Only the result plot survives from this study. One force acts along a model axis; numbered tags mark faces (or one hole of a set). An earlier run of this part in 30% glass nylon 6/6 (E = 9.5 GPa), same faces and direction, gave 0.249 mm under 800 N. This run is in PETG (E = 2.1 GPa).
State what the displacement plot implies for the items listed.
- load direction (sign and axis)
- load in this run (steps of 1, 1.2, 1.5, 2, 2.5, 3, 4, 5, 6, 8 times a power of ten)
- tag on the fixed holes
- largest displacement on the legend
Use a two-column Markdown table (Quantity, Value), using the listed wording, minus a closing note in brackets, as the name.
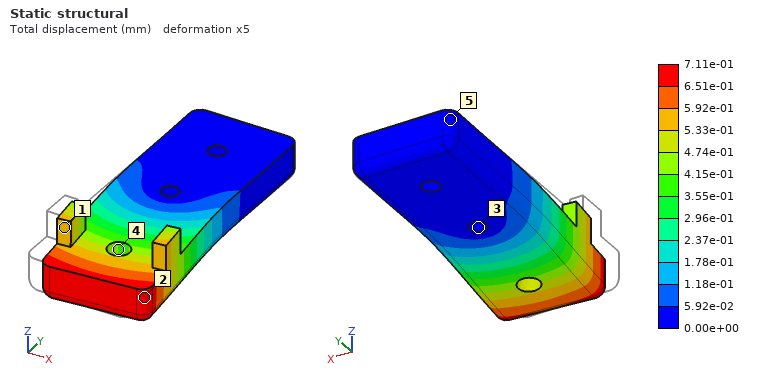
| Quantity | Value |
|---|---|
| load direction | +X |
| load in this run | 500 N |
| tag on the fixed holes | 3 |
| largest displacement on the legend | 7.11e-01 mm |
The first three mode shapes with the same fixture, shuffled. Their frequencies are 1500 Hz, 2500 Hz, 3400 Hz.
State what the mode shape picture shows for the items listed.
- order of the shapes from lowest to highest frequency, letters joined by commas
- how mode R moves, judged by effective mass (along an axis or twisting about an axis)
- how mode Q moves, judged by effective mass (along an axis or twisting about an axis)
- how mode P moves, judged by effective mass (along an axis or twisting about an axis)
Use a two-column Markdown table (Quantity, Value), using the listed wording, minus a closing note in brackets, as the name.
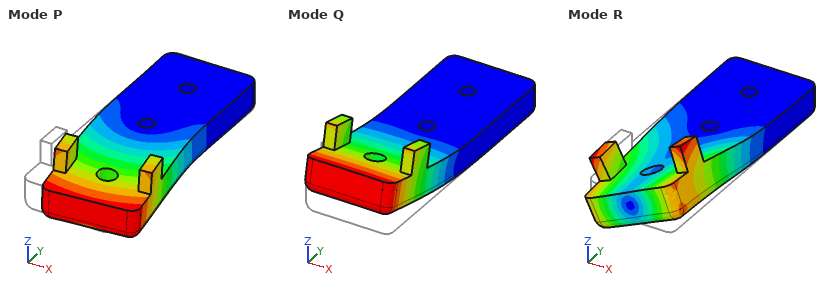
| Quantity | Value |
|---|---|
| order of the shapes from lowest to highest frequency, letters joined by commas | Q, P, R |
| how mode R moves, judged by effective mass | twisting about Y |
| how mode Q moves, judged by effective mass | along Z |
| how mode P moves, judged by effective mass | along X |
